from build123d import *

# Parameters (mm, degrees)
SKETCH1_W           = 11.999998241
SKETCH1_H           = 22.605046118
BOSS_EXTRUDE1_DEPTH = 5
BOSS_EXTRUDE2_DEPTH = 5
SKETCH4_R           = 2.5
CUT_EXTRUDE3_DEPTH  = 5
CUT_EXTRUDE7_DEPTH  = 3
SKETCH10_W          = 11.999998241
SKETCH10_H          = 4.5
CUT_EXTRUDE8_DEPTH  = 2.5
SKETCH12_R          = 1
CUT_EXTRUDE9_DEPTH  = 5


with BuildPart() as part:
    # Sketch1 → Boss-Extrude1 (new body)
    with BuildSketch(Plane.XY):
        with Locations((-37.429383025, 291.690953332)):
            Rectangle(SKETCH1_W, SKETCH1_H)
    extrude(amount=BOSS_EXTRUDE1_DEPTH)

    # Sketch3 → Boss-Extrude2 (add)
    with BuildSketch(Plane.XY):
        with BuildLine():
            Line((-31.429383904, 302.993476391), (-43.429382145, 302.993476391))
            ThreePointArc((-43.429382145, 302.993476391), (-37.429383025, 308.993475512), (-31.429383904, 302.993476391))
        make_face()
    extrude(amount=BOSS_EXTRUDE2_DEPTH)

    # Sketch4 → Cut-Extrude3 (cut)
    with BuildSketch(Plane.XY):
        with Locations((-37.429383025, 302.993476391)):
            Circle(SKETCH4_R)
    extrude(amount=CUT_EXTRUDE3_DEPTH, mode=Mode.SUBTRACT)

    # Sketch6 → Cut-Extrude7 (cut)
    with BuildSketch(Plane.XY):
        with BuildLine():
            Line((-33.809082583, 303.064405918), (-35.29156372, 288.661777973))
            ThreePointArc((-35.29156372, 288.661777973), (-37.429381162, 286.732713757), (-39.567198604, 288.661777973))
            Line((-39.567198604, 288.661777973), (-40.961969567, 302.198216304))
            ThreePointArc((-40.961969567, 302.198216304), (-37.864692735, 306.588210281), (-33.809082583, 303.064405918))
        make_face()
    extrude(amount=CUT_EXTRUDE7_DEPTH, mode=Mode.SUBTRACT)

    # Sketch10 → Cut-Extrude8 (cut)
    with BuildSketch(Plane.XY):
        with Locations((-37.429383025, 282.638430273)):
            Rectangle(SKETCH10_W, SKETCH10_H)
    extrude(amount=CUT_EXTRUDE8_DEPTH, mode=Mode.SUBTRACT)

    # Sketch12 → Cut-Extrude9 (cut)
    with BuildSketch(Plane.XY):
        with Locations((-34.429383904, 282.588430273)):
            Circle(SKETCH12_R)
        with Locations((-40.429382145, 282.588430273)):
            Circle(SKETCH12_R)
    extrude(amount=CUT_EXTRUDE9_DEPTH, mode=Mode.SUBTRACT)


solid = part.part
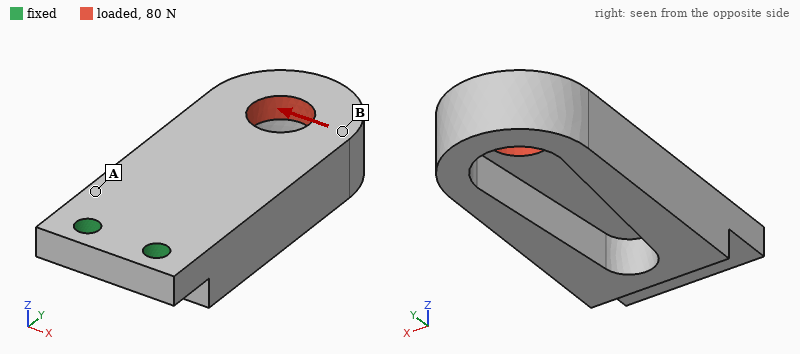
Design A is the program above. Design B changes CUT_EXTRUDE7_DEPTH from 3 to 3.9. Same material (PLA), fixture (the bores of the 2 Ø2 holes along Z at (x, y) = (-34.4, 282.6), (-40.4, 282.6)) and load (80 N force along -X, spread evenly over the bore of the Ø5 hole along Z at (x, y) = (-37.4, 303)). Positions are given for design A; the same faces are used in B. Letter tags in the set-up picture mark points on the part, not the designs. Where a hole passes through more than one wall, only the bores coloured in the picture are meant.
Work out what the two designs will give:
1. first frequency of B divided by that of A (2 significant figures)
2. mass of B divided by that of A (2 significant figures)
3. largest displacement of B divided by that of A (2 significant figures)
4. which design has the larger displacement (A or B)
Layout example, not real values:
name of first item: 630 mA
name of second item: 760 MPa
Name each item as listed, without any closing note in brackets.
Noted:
first frequency of B divided by that of A: 1.0
mass of B divided by that of A: 0.93
largest displacement of B divided by that of A: 1.1
which design has the larger displacement: B
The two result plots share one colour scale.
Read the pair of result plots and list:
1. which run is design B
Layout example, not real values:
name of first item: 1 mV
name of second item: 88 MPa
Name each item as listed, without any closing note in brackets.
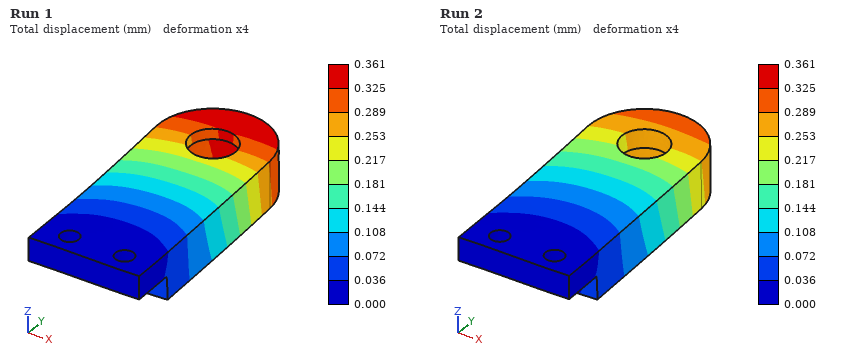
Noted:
which run is design B: Run 1
